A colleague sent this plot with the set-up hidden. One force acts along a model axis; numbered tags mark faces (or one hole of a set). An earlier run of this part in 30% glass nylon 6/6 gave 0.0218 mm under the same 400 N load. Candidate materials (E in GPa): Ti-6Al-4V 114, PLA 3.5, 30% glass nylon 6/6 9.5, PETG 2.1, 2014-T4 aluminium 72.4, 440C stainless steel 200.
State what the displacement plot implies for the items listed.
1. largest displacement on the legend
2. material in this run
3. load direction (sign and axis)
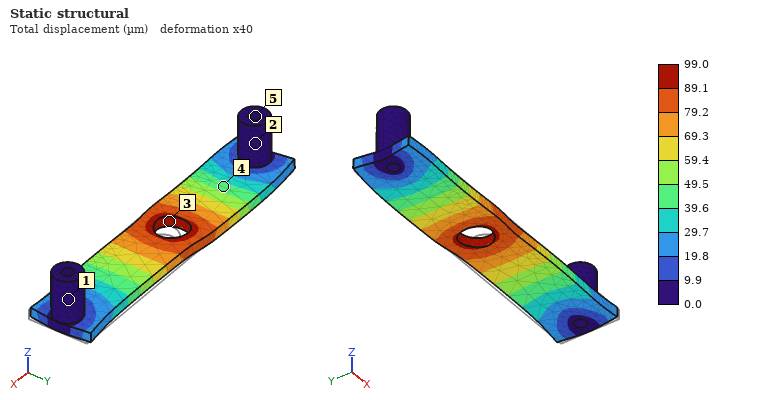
99.0 µm
PETG
-X
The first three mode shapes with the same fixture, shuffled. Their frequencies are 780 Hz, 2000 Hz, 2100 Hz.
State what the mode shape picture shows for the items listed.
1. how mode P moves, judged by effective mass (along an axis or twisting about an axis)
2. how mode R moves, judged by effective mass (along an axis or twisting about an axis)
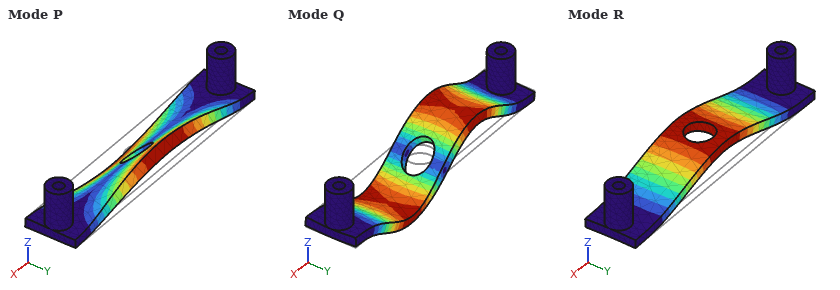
twisting about X
along Z
